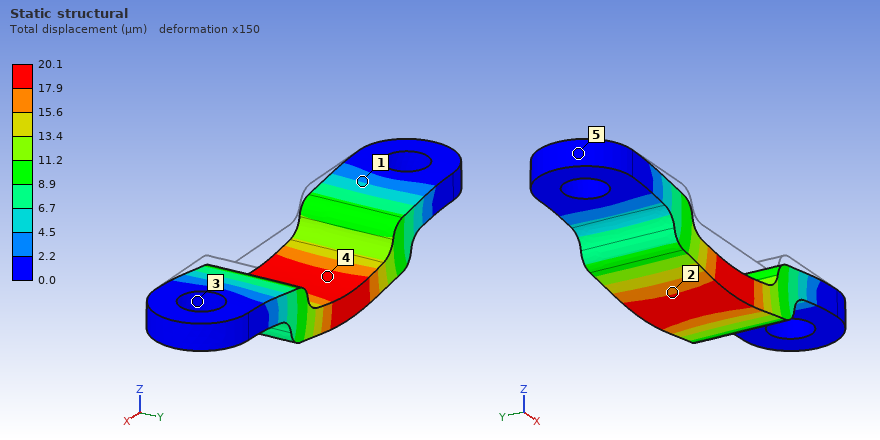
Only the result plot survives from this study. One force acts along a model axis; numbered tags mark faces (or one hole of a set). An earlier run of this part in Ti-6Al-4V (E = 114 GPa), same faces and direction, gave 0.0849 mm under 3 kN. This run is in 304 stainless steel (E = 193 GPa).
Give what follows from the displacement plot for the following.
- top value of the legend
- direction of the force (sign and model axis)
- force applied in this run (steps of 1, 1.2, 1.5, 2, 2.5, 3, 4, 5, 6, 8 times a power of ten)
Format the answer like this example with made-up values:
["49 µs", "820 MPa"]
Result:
["20.1 µm", "-Z", "1.2 kN"]
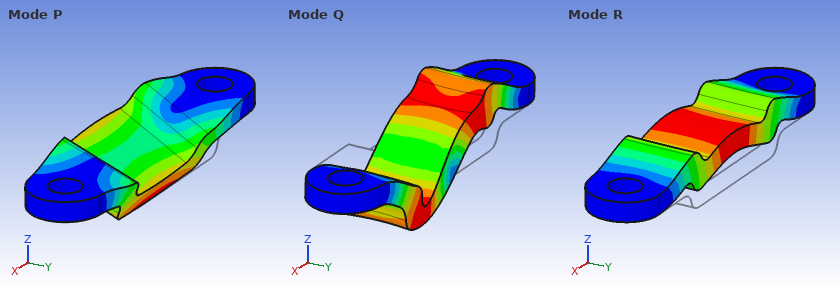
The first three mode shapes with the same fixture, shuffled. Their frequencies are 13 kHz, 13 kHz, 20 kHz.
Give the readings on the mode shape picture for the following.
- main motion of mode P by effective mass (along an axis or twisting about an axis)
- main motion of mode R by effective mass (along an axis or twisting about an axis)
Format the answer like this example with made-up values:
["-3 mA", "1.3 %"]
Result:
["along Y", "along Z"]
